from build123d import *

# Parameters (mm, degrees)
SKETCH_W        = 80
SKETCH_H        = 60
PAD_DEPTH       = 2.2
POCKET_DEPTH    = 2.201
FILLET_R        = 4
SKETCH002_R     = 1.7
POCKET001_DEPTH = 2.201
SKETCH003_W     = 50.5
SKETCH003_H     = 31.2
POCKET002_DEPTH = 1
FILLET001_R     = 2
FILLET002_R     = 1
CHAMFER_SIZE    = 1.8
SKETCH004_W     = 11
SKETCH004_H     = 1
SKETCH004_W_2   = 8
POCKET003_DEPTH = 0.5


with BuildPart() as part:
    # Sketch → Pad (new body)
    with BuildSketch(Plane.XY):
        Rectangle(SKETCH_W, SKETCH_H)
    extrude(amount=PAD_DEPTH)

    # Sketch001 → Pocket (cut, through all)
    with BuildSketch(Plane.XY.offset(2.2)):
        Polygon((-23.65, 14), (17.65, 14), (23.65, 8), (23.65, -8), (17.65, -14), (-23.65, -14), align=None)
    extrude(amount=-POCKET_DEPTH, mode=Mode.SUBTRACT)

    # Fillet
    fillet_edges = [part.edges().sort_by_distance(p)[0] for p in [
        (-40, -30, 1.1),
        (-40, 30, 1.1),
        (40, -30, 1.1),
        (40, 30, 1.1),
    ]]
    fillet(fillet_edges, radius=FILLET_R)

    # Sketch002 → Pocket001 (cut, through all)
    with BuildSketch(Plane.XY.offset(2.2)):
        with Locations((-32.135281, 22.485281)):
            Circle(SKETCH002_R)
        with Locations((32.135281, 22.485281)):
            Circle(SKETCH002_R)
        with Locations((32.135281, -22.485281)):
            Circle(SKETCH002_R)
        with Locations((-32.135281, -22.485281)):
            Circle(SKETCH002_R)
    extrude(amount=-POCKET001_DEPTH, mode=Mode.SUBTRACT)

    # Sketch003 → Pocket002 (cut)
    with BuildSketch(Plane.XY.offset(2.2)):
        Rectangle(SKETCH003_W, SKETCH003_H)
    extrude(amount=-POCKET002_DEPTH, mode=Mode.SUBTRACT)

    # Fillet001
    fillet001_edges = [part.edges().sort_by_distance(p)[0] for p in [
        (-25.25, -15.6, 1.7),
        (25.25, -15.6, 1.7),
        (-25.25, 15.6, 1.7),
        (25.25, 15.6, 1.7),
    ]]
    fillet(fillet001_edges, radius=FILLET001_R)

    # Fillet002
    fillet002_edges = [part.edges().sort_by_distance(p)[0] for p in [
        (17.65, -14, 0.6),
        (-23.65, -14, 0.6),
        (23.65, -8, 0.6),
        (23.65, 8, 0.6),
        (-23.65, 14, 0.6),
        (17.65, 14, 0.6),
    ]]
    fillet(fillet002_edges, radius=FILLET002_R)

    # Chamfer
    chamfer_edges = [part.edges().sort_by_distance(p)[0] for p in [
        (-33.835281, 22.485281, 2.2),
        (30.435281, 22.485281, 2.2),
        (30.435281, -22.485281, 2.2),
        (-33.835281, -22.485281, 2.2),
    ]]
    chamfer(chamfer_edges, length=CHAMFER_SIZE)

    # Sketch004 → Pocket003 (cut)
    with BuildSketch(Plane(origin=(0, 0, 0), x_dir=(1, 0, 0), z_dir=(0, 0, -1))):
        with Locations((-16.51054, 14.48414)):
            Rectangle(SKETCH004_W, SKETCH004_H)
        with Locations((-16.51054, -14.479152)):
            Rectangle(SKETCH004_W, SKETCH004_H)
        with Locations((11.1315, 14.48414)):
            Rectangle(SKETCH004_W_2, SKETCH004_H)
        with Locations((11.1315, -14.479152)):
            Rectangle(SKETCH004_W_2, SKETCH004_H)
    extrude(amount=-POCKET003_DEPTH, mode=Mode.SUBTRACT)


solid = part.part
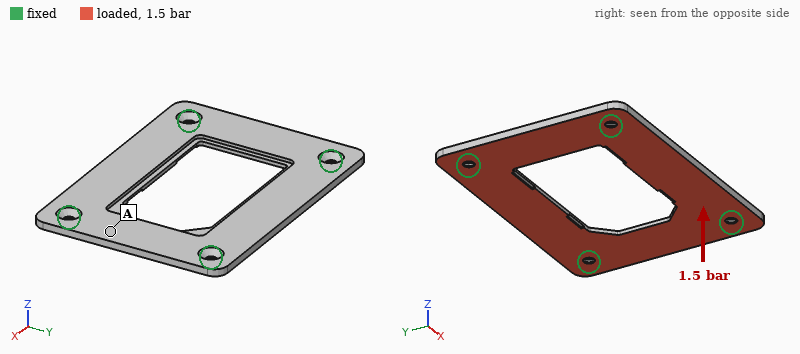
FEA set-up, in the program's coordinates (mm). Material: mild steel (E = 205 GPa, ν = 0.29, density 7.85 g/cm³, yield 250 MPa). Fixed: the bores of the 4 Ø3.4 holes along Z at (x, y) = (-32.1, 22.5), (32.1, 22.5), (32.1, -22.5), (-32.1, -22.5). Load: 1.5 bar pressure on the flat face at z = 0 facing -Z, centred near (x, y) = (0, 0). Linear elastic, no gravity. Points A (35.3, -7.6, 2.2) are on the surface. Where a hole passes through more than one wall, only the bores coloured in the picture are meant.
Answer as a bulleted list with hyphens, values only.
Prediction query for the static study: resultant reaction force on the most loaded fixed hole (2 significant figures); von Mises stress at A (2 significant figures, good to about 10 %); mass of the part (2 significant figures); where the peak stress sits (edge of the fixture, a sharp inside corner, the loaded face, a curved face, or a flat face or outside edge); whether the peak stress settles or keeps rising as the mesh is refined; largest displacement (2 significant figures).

- 290 N
- 20 MPa
- 57 g
- edge of the fixture
- keeps rising
- 61 µm
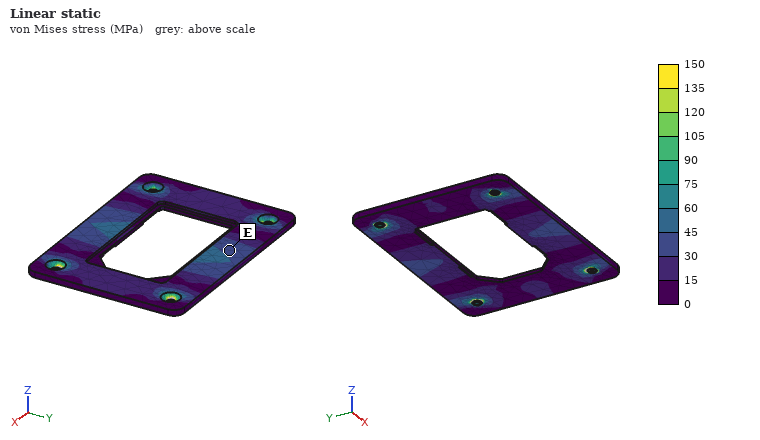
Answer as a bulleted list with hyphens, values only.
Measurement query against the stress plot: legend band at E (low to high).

- 30 to 45 MPa
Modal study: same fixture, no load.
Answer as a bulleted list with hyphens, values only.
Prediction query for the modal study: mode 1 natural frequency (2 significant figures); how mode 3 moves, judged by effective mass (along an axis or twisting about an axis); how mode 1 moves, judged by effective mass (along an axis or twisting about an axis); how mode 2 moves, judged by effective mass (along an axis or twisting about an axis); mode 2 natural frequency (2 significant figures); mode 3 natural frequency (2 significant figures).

- 2300 Hz
- along Z
- along Z
- twisting about X
- 2500 Hz
- 4200 Hz
